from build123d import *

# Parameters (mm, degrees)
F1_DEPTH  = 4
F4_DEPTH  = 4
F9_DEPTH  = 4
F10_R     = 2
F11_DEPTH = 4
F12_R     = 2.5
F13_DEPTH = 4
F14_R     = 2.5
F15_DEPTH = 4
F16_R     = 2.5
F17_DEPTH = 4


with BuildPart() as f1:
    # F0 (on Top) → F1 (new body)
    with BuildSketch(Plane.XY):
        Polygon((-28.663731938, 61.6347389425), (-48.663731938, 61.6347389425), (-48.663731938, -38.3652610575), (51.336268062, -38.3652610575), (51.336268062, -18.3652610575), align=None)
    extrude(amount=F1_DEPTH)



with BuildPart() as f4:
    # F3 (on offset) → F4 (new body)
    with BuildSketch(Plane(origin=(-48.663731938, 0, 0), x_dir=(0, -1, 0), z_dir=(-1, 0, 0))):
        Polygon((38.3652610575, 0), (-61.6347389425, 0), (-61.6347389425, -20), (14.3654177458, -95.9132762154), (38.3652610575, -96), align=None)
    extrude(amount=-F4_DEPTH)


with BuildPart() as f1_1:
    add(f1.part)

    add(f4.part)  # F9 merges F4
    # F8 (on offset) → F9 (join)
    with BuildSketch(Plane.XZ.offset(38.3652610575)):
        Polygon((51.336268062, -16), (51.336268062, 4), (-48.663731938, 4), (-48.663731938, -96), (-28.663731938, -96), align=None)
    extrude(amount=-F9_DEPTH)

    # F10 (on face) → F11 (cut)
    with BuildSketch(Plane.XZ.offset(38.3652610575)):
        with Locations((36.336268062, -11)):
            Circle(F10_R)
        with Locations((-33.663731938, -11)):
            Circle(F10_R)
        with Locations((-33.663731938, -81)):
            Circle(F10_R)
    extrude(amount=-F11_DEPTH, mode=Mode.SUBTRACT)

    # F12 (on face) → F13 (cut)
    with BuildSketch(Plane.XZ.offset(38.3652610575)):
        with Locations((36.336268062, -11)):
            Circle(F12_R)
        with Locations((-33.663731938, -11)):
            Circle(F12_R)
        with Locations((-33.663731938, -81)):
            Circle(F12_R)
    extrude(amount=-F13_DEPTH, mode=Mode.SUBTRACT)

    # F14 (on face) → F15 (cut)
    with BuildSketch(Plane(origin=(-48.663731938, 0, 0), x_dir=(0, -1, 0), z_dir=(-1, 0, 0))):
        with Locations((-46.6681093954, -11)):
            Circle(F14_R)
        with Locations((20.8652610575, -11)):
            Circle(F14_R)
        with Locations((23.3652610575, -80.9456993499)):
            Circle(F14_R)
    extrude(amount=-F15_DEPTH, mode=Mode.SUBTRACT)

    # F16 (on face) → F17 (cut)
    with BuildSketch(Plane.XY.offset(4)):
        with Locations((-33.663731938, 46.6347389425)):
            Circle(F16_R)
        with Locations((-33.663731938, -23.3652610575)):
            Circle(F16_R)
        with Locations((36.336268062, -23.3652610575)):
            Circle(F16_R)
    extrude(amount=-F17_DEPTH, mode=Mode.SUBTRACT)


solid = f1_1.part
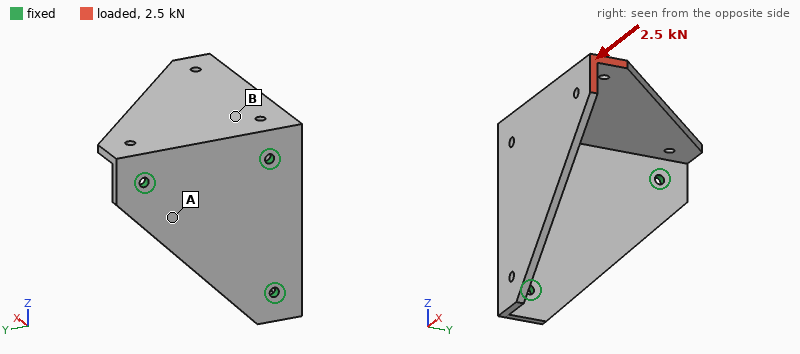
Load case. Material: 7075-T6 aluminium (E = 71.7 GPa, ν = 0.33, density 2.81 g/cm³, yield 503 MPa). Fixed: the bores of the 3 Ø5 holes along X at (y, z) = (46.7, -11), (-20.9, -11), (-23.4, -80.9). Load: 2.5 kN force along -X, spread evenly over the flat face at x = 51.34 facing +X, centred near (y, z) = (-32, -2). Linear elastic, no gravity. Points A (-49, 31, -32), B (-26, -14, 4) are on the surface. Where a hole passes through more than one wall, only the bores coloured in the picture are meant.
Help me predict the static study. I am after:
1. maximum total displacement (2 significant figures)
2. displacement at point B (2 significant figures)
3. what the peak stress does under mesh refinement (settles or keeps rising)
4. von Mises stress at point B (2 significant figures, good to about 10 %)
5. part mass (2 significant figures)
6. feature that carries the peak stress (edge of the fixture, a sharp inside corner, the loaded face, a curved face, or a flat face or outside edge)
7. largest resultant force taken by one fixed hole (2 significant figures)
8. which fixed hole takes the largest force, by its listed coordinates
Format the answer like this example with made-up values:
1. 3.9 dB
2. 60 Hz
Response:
1. 0.22 mm
2. 0.079 mm
3. keeps rising
4. 19 MPa
5. 220 g
6. edge of the fixture
7. 3.0 kN
8. (-20.9, -11)
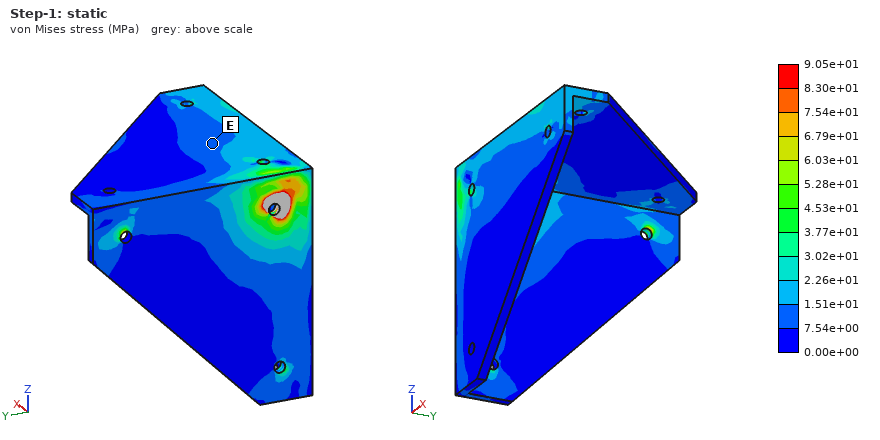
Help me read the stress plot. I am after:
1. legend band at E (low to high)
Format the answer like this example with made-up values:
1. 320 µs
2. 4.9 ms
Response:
1. 7.54e+00 to 1.51e+01 MPa
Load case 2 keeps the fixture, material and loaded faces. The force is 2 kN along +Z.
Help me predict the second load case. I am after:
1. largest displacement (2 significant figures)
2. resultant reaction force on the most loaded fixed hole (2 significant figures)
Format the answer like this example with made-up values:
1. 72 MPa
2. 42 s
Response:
1. 0.77 mm
2. 3.0 kN
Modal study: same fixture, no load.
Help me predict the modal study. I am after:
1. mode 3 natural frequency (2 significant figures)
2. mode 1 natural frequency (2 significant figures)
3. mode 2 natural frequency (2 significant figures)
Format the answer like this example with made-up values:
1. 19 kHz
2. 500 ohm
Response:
1. 1900 Hz
2. 1000 Hz
3. 1600 Hz
